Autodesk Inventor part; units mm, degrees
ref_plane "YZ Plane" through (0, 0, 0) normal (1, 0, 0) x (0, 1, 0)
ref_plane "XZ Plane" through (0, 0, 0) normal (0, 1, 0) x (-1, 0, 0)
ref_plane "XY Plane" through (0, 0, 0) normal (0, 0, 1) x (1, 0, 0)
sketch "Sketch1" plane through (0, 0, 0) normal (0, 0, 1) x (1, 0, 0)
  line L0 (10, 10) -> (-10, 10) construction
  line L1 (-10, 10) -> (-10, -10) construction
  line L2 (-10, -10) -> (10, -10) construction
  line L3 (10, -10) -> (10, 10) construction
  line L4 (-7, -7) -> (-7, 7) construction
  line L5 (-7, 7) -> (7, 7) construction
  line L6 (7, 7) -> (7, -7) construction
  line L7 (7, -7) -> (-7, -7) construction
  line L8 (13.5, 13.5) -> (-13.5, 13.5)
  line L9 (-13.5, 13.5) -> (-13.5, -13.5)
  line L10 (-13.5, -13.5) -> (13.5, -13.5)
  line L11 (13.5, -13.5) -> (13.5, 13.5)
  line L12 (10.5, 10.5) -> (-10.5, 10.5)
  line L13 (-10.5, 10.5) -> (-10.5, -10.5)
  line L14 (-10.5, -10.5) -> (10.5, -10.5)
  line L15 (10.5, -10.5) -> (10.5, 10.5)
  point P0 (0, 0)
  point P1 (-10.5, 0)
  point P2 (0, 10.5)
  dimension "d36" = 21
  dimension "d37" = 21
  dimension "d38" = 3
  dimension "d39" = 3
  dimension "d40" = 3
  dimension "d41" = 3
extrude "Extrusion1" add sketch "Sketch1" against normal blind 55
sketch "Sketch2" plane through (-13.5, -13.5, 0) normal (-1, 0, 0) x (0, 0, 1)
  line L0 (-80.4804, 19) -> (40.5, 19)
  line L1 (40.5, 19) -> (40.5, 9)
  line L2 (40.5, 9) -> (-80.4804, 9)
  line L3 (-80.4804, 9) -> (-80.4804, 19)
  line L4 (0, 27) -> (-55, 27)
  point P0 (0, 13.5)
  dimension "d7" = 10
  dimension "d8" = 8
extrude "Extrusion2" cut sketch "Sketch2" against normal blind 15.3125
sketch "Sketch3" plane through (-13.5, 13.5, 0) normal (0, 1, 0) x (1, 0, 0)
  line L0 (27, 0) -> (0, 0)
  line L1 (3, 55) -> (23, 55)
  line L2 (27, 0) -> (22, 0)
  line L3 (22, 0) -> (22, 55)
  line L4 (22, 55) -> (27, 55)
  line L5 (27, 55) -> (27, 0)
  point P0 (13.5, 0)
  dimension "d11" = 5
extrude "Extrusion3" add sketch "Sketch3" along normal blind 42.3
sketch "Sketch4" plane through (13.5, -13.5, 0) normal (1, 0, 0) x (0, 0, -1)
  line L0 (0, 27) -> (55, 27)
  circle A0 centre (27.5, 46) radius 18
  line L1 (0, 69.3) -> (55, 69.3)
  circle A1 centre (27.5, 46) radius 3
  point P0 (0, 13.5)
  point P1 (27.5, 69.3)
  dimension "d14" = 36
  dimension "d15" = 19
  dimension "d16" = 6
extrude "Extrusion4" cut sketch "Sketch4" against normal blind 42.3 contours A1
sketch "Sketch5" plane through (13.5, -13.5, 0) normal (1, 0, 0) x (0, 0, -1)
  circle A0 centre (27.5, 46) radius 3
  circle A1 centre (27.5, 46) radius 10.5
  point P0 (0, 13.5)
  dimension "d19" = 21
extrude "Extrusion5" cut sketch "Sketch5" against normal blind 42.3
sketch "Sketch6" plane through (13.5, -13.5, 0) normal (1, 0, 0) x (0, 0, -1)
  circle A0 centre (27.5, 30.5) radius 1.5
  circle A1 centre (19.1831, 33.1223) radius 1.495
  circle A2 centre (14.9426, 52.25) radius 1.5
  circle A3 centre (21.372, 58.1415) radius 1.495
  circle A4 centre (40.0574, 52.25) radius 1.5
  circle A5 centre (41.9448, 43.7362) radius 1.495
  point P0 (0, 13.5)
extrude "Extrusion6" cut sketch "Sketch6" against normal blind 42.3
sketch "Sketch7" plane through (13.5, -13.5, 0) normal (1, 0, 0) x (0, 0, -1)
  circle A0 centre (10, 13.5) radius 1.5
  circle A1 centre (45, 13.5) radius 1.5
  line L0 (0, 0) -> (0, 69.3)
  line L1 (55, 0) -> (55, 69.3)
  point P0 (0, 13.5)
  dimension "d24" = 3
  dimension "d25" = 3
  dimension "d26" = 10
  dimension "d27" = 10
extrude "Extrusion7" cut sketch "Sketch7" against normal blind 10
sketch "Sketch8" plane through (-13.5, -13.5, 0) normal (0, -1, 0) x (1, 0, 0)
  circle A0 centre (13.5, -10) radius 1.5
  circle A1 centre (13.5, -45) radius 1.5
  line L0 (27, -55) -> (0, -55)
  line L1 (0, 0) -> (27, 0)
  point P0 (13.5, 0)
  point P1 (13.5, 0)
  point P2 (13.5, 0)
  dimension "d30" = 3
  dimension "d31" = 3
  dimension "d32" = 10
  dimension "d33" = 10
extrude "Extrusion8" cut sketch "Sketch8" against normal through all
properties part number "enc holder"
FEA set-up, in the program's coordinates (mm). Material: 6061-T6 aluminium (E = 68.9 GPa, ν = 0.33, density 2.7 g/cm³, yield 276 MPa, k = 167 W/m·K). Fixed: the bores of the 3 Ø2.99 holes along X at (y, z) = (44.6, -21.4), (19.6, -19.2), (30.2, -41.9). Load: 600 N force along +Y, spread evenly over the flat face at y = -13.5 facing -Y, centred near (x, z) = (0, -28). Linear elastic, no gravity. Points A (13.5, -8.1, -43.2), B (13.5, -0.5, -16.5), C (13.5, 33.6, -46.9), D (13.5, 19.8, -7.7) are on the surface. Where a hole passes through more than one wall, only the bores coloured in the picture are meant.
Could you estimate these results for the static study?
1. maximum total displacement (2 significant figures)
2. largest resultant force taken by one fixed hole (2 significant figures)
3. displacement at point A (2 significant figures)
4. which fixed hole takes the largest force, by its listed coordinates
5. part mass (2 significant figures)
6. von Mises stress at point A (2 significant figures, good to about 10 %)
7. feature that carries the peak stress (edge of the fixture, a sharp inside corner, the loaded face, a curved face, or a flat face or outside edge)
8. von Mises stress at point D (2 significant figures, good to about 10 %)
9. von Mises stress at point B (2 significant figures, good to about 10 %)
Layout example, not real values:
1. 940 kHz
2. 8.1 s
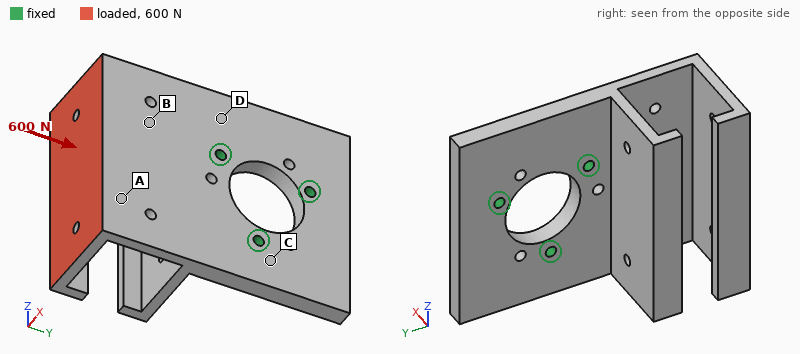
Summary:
1. 0.73 mm
2. 330 N
3. 0.23 mm
4. (19.6, -19.2)
5. 64 g
6. 72 MPa
7. a curved face
8. 17 MPa
9. 80 MPa
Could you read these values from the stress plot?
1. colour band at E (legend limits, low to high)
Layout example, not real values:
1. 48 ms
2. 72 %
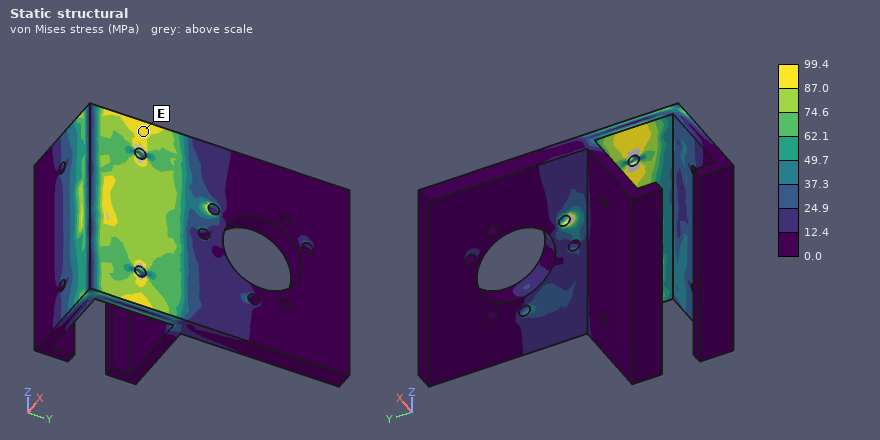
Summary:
1. 87.0 to 99.4 MPa
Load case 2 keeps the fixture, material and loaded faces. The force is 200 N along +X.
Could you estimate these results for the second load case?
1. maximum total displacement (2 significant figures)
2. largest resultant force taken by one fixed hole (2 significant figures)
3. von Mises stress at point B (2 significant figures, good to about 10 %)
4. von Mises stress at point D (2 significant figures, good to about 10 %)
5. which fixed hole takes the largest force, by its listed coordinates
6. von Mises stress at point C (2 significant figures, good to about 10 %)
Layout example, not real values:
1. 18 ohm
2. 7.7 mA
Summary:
1. 0.32 mm
2. 270 N
3. 31 MPa
4. 17 MPa
5. (19.6, -19.2)
6. 8.8 MPa
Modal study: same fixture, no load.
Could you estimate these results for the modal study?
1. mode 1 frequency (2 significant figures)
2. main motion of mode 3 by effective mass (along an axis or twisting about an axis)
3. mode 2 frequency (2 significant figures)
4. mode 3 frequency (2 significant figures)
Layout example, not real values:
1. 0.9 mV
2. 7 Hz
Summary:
1. 1000 Hz
2. along X
3. 1600 Hz
4. 2400 Hz
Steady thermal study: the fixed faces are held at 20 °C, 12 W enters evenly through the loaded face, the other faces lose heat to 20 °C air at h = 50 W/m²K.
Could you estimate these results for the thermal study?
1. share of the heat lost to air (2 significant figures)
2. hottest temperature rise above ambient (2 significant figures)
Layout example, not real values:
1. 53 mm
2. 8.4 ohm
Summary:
1. 29 %
2. 15 K
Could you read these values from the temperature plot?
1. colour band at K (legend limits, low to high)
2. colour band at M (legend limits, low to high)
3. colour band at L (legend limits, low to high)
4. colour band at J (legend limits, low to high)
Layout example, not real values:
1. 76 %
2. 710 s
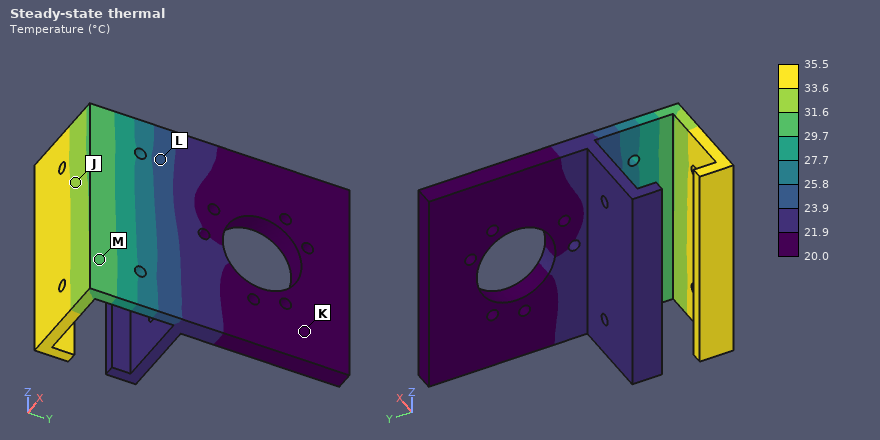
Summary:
1. 20.0 to 21.9 °C
2. 29.7 to 31.6 °C
3. 23.9 to 25.8 °C
4. 31.6 to 33.6 °C
